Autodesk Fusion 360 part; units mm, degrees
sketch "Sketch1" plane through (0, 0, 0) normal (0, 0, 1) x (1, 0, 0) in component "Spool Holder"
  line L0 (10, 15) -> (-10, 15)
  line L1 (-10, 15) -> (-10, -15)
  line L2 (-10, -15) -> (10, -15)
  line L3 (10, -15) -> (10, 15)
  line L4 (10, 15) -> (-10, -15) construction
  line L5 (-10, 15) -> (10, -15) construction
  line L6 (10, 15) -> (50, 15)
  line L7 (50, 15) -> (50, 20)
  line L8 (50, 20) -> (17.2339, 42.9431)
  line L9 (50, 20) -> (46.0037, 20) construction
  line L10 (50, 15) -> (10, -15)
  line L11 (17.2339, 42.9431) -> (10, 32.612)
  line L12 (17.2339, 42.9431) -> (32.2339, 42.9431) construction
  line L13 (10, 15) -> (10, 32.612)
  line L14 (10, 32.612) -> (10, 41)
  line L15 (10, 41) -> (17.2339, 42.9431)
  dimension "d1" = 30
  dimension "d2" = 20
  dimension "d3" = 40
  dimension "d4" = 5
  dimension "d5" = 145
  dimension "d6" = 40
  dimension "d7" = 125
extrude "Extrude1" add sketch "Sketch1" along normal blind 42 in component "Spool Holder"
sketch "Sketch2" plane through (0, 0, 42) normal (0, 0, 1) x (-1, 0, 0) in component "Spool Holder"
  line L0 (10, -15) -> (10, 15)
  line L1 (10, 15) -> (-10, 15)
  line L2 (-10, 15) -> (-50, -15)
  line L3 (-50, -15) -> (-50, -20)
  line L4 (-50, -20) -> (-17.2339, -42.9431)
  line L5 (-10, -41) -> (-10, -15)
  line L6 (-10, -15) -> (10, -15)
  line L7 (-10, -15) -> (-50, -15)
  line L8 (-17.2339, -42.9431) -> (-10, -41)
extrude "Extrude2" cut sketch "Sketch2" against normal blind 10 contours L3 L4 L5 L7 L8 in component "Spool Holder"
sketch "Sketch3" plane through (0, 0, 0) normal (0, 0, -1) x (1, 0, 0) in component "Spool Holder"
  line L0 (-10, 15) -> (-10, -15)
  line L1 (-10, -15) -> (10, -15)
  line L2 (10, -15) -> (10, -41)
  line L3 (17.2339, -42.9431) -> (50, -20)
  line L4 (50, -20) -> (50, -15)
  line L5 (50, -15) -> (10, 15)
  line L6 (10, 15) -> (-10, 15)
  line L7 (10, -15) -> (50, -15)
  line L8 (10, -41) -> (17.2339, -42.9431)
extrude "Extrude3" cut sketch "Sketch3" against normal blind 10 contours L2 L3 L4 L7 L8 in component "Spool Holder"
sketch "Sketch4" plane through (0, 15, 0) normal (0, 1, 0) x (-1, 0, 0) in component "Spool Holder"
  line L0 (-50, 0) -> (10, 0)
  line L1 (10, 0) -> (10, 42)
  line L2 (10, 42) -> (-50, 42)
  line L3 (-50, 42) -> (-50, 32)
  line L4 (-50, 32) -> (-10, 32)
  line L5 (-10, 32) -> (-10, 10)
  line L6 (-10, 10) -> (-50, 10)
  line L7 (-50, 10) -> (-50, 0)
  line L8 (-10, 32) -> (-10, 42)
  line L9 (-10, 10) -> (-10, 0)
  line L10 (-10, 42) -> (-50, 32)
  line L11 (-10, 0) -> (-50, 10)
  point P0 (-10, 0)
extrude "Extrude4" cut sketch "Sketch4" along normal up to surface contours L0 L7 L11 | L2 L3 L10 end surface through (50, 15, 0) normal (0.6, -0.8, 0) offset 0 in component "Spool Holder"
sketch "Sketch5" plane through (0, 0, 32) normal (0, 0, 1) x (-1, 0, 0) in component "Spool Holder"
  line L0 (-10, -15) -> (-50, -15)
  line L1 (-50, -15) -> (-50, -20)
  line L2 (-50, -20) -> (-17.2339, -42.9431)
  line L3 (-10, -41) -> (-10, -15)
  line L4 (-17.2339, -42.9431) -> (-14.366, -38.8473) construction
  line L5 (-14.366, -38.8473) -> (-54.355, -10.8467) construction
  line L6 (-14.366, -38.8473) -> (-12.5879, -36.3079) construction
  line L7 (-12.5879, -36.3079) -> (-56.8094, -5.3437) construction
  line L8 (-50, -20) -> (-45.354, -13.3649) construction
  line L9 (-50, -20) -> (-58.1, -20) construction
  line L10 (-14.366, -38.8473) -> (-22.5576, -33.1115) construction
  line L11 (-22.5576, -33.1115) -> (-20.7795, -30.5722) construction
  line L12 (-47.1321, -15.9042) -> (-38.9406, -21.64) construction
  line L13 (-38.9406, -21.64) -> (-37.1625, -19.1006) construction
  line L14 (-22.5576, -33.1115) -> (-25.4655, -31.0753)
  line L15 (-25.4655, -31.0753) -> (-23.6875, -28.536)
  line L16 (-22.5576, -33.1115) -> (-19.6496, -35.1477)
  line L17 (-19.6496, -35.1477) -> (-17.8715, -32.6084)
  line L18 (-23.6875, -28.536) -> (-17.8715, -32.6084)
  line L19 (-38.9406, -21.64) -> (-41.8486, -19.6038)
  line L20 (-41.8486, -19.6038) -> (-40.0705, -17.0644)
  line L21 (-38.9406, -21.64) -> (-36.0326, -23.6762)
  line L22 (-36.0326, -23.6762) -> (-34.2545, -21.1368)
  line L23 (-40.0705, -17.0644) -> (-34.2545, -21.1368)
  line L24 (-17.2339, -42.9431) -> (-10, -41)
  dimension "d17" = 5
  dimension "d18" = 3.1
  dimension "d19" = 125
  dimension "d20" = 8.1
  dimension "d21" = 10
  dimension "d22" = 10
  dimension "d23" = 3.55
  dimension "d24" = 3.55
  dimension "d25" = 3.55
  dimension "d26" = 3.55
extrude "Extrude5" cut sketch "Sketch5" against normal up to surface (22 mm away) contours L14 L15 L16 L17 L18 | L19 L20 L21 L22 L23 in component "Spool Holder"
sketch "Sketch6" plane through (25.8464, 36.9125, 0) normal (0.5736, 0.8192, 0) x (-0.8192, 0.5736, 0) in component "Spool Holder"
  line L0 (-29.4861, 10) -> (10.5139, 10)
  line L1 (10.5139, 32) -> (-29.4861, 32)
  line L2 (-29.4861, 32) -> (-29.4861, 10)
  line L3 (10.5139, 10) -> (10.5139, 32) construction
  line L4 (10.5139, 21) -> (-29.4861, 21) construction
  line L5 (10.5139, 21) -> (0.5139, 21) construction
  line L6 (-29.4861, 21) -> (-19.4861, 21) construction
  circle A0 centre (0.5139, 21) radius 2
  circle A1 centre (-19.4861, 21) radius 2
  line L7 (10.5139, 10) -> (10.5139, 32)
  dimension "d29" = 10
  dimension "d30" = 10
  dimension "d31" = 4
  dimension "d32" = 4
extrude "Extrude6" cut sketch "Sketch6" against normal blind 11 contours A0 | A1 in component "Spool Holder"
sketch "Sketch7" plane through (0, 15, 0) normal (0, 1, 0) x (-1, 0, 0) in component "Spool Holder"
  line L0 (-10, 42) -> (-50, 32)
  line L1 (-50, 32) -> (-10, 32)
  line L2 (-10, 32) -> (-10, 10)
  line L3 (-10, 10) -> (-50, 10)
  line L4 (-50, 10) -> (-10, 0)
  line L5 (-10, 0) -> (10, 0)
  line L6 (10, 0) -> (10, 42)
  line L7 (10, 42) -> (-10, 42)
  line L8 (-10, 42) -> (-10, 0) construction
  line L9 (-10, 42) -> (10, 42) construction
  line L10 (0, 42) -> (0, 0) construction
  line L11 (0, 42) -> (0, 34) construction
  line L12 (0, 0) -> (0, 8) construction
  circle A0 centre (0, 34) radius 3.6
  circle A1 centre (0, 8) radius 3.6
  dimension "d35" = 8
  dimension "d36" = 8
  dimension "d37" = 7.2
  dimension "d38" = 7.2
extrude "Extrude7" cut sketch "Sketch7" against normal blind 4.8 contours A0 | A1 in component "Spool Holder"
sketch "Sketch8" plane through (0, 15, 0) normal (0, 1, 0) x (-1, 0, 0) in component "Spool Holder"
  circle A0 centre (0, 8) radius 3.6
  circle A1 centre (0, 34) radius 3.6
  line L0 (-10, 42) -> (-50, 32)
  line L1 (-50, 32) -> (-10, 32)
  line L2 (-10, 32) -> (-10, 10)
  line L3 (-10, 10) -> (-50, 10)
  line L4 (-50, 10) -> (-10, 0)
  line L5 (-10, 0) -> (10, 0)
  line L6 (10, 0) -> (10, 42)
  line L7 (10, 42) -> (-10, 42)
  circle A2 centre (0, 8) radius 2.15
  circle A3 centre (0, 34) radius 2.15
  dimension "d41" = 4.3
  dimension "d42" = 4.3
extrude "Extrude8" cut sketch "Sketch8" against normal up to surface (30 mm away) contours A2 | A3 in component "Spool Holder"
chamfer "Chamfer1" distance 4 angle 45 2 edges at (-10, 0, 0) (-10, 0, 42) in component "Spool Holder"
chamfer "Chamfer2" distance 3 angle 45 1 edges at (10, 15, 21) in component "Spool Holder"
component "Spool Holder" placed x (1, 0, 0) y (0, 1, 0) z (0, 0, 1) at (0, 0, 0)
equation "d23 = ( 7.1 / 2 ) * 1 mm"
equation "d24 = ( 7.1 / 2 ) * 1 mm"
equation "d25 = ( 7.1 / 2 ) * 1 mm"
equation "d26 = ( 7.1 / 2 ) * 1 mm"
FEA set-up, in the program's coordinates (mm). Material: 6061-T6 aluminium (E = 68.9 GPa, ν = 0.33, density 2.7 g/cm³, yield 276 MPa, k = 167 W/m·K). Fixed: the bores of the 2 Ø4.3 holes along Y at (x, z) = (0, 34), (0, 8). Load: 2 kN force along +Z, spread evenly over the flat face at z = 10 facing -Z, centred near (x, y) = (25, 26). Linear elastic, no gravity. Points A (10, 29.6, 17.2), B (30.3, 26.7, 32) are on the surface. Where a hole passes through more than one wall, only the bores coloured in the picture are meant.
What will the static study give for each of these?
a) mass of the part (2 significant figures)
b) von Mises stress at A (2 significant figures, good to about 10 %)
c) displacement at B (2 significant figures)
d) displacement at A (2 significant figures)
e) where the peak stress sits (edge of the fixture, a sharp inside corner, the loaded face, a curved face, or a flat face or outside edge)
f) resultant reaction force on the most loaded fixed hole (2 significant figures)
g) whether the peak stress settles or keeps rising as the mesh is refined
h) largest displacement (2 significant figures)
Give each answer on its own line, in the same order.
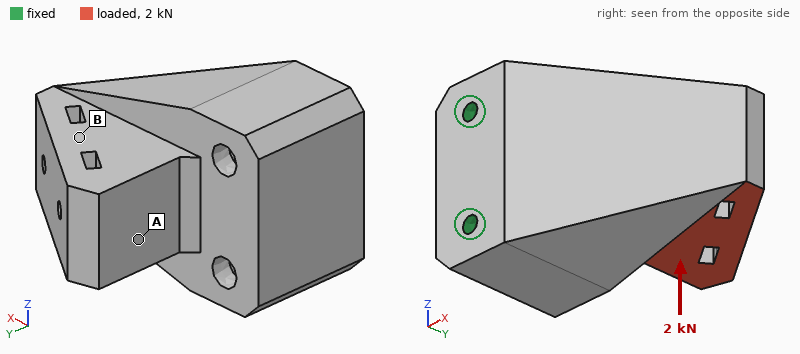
160 g
5.0 MPa
11 µm
9.7 µm
edge of the fixture
2.5 kN
keeps rising
16 µm
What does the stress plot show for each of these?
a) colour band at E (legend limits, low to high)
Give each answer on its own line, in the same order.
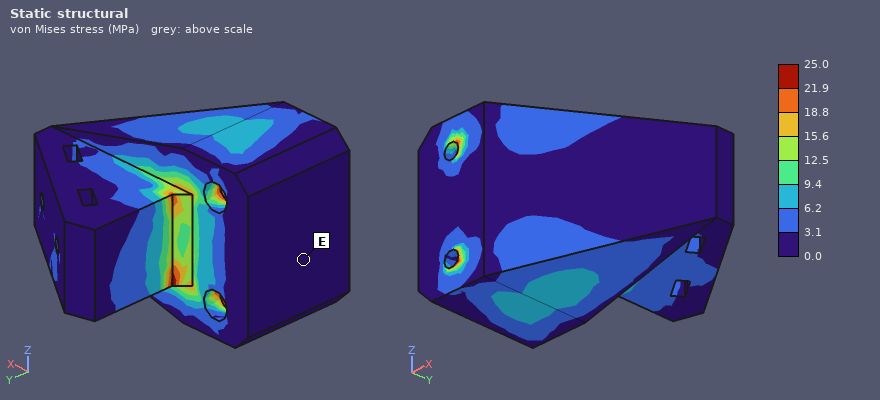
0.0 to 3.1 MPa
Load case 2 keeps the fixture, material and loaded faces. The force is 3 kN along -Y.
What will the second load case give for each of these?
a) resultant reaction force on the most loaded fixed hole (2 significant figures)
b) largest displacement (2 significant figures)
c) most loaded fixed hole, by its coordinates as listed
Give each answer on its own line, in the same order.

2.4 kN
27 µm
(0, 8)
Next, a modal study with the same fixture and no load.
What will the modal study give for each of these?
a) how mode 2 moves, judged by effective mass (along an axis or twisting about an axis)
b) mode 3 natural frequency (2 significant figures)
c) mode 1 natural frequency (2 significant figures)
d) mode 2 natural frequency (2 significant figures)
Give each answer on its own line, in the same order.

along Z
15 kHz
7000 Hz
9700 Hz
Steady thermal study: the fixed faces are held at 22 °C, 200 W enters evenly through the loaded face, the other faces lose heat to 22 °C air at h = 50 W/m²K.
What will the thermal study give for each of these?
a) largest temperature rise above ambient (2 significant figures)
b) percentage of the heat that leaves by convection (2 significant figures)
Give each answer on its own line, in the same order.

68 K
6.4 %
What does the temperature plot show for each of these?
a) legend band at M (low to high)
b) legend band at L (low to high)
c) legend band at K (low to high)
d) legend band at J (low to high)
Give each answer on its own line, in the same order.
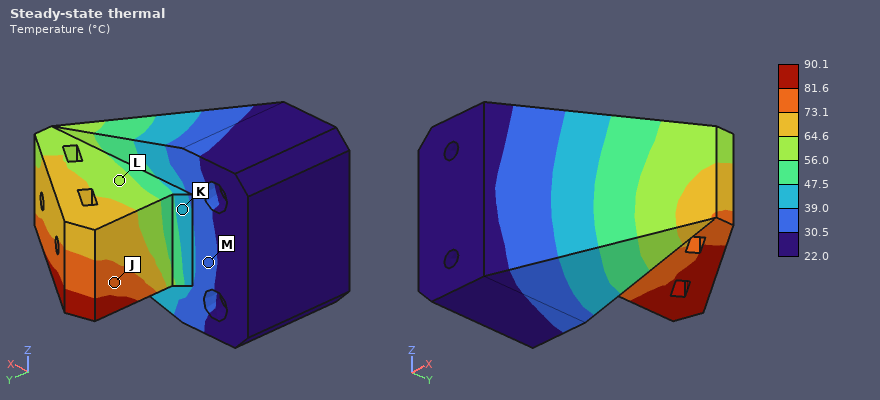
30.5 to 39.0 °C
56.0 to 64.6 °C
39.0 to 47.5 °C
73.1 to 81.6 °C
